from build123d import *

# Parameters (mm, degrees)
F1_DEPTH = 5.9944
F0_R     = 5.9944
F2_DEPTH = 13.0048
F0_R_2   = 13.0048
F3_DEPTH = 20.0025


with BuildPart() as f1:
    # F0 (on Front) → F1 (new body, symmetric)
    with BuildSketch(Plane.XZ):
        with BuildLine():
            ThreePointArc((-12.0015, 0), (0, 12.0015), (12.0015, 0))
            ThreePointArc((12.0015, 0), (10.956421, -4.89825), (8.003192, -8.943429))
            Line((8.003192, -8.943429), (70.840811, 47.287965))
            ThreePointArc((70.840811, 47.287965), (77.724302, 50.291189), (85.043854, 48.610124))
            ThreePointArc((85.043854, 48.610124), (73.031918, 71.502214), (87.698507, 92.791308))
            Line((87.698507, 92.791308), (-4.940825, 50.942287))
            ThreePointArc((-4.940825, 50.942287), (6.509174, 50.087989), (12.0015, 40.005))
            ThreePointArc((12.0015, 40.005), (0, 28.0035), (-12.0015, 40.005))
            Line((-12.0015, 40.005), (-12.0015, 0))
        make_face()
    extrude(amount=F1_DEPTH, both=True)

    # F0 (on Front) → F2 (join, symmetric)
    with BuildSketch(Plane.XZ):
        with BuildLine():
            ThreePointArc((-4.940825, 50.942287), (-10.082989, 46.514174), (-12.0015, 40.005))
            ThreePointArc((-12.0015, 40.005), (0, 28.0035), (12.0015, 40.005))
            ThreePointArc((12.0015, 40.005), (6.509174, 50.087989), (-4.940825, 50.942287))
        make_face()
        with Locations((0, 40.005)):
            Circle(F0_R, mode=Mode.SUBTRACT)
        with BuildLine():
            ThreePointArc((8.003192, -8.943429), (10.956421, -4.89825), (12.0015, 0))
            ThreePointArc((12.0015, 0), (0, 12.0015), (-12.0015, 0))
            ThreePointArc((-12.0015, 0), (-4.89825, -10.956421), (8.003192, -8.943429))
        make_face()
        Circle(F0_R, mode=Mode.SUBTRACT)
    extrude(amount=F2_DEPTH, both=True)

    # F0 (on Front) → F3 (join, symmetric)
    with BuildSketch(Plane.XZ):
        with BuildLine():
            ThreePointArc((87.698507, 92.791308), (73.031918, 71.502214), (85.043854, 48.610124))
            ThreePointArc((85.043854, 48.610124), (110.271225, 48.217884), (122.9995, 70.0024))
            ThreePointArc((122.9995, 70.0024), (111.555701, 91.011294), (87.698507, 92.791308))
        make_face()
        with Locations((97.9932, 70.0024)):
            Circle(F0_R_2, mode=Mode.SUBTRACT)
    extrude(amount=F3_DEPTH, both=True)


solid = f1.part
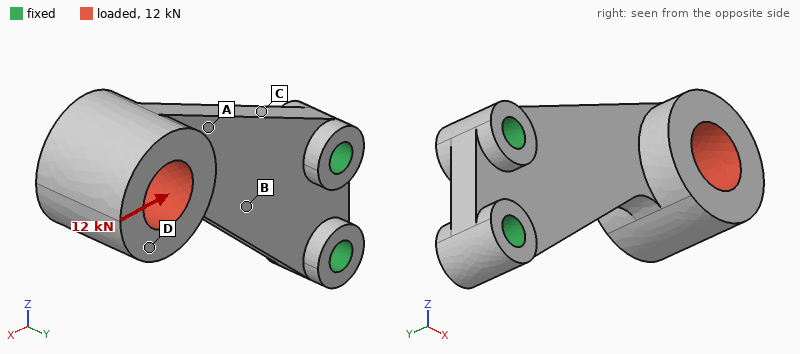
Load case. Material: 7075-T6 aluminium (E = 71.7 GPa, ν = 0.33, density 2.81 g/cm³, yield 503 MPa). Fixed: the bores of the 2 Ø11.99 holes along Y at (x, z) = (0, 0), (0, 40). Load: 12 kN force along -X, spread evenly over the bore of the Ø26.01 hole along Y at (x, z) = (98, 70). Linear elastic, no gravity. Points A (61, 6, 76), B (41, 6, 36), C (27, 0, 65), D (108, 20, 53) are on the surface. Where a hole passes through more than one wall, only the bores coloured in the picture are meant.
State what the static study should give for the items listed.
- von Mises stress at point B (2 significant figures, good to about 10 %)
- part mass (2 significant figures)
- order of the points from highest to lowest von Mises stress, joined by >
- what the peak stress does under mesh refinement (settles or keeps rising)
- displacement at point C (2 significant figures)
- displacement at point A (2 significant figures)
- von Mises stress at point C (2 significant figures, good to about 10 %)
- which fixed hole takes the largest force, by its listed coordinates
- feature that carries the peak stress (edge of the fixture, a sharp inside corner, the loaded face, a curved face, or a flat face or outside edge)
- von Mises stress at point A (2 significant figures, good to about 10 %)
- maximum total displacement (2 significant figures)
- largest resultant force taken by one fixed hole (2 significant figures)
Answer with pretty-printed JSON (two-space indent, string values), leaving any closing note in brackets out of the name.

{
  "von Mises stress at point B": "26 MPa",
  "part mass": "340 g",
  "order of the points from highest to lowest von Mises stress, joined by >": "C > A > B > D",
  "what the peak stress does under mesh refinement": "keeps rising",
  "displacement at point C": "0.065 mm",
  "displacement at point A": "0.16 mm",
  "von Mises stress at point C": "95 MPa",
  "which fixed hole takes the largest force, by its listed coordinates": "(0, 40)",
  "feature that carries the peak stress": "edge of the fixture",
  "von Mises stress at point A": "49 MPa",
  "maximum total displacement": "0.34 mm",
  "largest resultant force taken by one fixed hole": "19 kN"
}
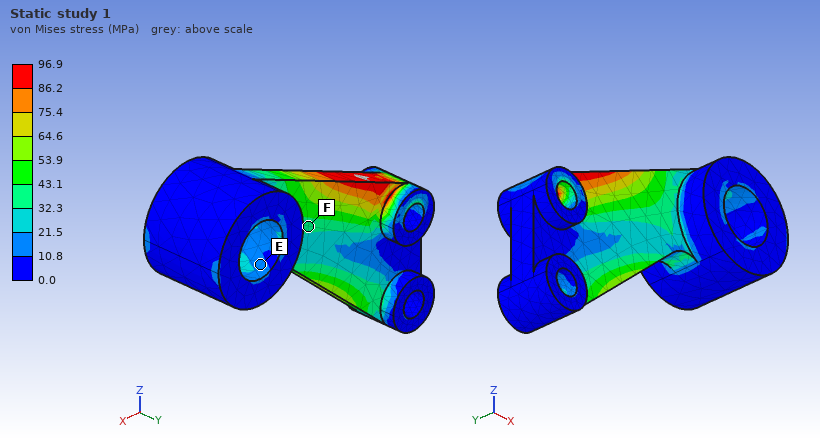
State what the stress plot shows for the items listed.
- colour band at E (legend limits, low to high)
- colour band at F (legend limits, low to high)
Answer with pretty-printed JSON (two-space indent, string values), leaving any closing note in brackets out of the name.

{
  "colour band at E": "10.8 to 21.5 MPa",
  "colour band at F": "32.3 to 43.1 MPa"
}
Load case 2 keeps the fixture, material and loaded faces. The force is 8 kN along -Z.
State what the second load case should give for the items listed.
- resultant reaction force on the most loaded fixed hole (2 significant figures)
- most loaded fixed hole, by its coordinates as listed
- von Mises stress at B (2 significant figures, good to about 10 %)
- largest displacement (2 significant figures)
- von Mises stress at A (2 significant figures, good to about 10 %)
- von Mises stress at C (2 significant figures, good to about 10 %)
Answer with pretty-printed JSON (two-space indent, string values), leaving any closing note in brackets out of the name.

{
  "resultant reaction force on the most loaded fixed hole": "19 kN",
  "most loaded fixed hole, by its coordinates as listed": "(0, 0)",
  "von Mises stress at B": "75 MPa",
  "largest displacement": "0.65 mm",
  "von Mises stress at A": "67 MPa",
  "von Mises stress at C": "120 MPa"
}
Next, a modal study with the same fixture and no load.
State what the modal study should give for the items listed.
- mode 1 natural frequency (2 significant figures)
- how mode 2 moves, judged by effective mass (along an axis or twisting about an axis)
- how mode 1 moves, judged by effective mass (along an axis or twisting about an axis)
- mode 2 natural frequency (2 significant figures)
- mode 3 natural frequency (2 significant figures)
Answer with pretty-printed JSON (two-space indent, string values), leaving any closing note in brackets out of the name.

{
  "mode 1 natural frequency": "460 Hz",
  "how mode 2 moves, judged by effective mass": "along Z",
  "how mode 1 moves, judged by effective mass": "along Y",
  "mode 2 natural frequency": "1500 Hz",
  "mode 3 natural frequency": "1800 Hz"
}
